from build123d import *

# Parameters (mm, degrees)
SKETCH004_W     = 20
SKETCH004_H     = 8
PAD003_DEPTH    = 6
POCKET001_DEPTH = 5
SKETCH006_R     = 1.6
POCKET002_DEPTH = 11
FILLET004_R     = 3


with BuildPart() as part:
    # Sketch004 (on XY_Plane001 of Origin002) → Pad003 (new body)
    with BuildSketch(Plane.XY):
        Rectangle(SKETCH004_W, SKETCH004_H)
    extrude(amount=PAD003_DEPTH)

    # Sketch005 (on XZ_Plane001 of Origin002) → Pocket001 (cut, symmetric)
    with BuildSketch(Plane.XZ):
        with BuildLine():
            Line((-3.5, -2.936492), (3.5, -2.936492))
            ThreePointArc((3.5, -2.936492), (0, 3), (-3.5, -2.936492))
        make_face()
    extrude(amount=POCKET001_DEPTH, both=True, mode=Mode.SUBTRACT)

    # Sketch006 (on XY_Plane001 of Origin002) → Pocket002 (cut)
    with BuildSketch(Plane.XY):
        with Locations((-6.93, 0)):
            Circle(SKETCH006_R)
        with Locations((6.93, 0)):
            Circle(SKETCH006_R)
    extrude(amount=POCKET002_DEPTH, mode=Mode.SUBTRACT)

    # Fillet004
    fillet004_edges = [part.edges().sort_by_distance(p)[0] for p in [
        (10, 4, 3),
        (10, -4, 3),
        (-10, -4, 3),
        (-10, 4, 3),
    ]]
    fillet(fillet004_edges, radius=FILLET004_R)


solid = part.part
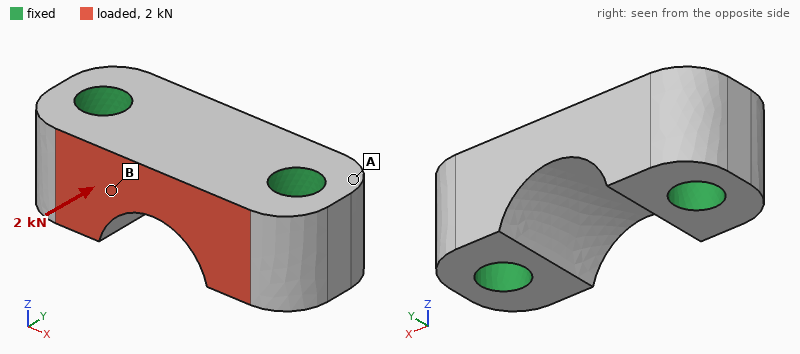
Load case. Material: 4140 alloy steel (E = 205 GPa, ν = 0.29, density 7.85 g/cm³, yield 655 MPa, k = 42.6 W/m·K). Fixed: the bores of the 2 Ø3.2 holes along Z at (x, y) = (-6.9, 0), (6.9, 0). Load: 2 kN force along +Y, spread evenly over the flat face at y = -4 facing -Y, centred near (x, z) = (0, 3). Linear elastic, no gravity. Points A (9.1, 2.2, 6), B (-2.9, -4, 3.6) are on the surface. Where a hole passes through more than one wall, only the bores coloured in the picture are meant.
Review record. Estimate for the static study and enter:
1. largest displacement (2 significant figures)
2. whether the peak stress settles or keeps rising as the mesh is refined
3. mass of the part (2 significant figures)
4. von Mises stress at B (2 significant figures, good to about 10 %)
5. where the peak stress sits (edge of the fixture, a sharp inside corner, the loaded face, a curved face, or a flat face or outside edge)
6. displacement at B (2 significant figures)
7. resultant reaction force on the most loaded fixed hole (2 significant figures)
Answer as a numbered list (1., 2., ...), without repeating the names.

1. 1.9 µm
2. keeps rising
3. 5.3 g
4. 30 MPa
5. edge of the fixture
6. 1.3 µm
7. 1.0 kN
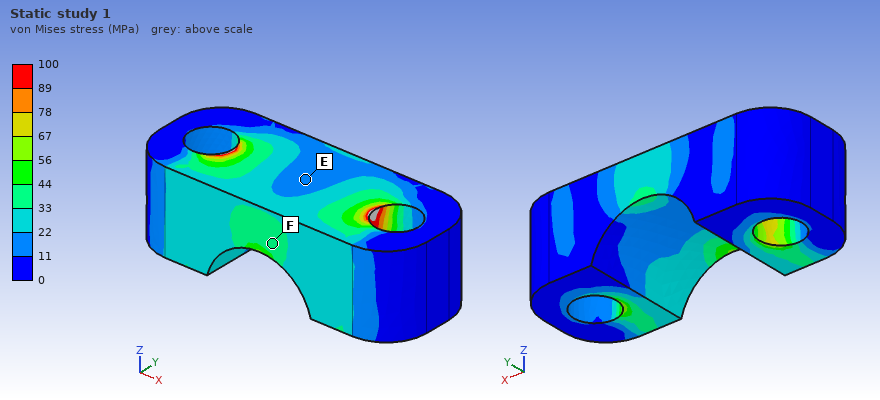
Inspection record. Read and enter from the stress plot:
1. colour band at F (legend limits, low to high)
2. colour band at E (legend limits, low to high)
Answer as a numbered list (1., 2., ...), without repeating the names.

1. 33 to 44 MPa
2. 11 to 22 MPa
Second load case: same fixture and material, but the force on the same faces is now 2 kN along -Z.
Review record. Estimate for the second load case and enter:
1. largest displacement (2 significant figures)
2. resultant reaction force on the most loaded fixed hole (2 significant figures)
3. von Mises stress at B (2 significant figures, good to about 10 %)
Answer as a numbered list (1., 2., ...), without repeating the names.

1. 5.2 µm
2. 1.0 kN
3. 100 MPa
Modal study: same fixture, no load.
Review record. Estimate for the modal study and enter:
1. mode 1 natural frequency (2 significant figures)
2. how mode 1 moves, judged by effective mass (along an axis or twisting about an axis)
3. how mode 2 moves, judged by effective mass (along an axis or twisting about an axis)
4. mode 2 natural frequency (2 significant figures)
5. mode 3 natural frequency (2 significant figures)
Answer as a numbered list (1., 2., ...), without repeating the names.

1. 110 kHz
2. along Y
3. along Z
4. 110 kHz
5. 140 kHz
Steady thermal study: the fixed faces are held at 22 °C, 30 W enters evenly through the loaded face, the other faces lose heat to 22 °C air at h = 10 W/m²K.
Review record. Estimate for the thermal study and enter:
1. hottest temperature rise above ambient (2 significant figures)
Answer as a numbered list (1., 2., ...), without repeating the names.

1. 50 K
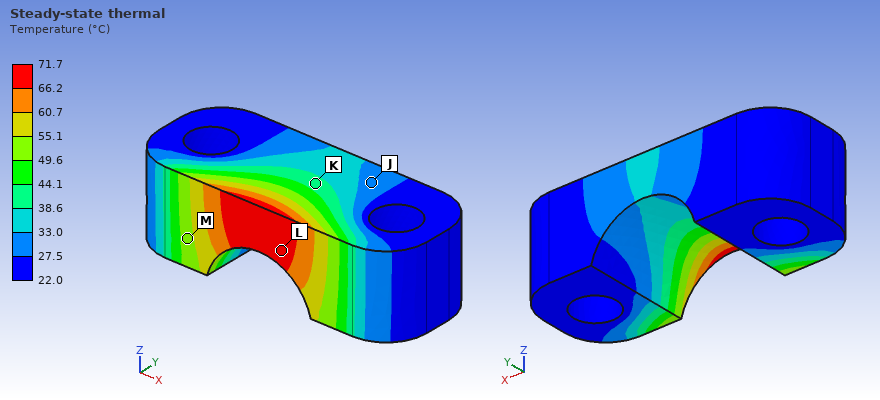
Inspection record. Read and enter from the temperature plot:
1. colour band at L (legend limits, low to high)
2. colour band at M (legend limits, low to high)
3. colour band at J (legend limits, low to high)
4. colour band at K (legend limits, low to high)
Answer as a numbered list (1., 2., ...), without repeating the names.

1. 66.2 to 71.7 °C
2. 49.6 to 55.1 °C
3. 27.5 to 33.0 °C
4. 38.6 to 44.1 °C
